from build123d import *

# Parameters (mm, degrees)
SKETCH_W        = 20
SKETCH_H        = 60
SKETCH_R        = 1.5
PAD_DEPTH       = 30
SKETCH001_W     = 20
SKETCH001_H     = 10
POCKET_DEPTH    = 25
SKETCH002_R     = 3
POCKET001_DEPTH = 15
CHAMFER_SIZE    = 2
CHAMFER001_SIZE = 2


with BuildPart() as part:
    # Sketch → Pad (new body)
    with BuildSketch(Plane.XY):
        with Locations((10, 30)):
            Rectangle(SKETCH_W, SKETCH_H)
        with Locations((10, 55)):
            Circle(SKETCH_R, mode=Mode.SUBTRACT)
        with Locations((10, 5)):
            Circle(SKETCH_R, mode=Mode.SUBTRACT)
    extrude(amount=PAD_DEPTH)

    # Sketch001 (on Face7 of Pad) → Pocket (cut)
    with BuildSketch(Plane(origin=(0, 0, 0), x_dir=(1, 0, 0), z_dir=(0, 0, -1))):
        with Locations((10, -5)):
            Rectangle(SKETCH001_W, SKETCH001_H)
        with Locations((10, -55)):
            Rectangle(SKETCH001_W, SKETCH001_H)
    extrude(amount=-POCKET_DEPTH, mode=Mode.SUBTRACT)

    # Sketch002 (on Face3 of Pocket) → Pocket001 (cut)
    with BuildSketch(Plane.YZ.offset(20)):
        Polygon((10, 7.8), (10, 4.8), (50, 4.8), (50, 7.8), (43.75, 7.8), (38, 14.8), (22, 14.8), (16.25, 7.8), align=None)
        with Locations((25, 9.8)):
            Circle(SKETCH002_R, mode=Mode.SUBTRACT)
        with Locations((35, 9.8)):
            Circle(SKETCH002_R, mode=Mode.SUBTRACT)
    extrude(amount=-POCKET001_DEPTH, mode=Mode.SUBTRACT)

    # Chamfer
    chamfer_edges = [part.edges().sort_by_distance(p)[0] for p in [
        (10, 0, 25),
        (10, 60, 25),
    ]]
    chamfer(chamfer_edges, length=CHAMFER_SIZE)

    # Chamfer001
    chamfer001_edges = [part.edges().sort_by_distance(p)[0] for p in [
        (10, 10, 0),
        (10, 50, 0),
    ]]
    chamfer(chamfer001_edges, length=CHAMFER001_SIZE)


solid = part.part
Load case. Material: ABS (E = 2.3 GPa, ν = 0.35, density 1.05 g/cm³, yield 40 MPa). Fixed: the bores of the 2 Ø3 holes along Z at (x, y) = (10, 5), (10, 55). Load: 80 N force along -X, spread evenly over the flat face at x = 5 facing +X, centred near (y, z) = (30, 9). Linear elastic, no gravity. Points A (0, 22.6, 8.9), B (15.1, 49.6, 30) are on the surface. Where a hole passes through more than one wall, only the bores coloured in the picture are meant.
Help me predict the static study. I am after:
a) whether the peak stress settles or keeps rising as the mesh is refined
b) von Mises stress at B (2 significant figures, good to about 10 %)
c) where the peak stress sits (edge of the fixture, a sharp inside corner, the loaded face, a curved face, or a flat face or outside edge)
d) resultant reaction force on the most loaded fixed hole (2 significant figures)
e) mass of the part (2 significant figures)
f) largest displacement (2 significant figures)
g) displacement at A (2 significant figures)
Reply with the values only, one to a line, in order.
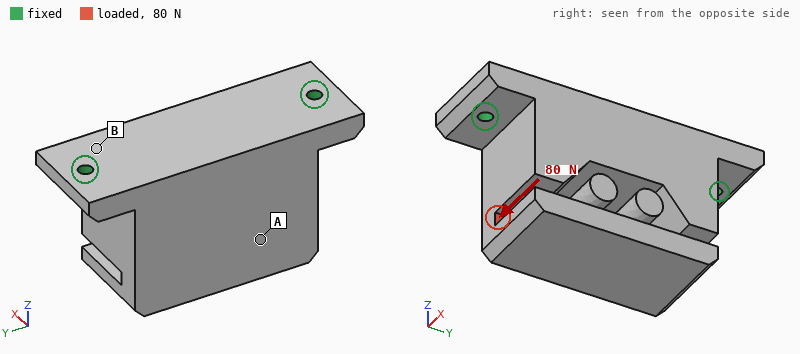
keeps rising
2.8 MPa
edge of the fixture
40 N
24 g
0.30 mm
0.21 mm
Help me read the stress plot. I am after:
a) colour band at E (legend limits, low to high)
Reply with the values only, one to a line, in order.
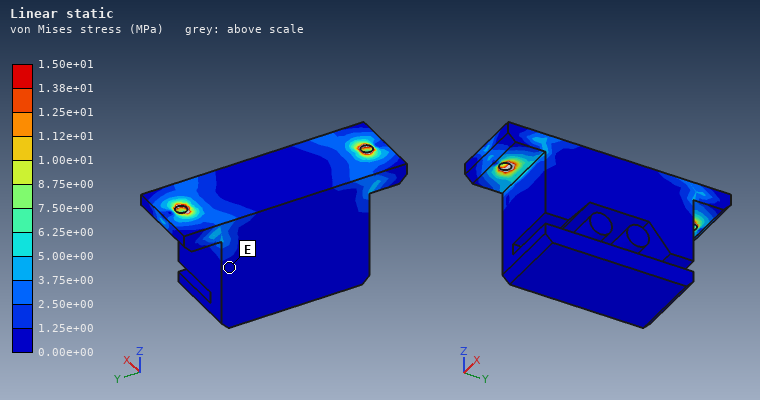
0.00e+00 to 1.25e+00 MPa
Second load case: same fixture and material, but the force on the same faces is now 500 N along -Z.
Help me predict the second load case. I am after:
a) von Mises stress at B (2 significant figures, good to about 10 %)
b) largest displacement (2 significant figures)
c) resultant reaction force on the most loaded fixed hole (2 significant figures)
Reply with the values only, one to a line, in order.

5.3 MPa
0.44 mm
280 N
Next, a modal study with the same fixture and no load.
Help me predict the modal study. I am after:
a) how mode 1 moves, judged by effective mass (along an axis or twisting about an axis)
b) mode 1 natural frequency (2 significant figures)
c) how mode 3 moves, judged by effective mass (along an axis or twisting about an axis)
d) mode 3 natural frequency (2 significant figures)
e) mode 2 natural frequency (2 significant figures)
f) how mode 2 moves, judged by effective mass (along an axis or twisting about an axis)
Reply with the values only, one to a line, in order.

along X
850 Hz
along Y
2700 Hz
2200 Hz
along Z
